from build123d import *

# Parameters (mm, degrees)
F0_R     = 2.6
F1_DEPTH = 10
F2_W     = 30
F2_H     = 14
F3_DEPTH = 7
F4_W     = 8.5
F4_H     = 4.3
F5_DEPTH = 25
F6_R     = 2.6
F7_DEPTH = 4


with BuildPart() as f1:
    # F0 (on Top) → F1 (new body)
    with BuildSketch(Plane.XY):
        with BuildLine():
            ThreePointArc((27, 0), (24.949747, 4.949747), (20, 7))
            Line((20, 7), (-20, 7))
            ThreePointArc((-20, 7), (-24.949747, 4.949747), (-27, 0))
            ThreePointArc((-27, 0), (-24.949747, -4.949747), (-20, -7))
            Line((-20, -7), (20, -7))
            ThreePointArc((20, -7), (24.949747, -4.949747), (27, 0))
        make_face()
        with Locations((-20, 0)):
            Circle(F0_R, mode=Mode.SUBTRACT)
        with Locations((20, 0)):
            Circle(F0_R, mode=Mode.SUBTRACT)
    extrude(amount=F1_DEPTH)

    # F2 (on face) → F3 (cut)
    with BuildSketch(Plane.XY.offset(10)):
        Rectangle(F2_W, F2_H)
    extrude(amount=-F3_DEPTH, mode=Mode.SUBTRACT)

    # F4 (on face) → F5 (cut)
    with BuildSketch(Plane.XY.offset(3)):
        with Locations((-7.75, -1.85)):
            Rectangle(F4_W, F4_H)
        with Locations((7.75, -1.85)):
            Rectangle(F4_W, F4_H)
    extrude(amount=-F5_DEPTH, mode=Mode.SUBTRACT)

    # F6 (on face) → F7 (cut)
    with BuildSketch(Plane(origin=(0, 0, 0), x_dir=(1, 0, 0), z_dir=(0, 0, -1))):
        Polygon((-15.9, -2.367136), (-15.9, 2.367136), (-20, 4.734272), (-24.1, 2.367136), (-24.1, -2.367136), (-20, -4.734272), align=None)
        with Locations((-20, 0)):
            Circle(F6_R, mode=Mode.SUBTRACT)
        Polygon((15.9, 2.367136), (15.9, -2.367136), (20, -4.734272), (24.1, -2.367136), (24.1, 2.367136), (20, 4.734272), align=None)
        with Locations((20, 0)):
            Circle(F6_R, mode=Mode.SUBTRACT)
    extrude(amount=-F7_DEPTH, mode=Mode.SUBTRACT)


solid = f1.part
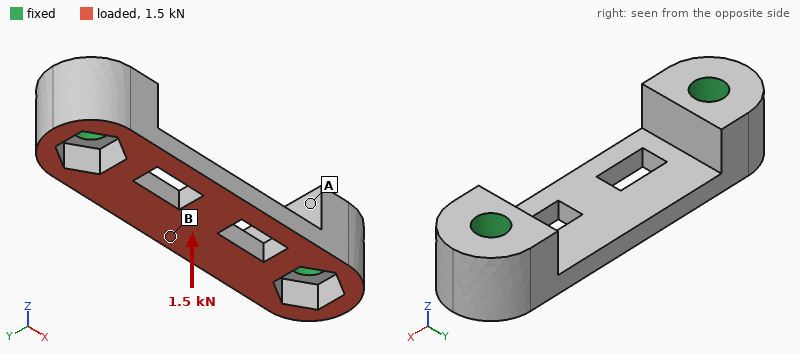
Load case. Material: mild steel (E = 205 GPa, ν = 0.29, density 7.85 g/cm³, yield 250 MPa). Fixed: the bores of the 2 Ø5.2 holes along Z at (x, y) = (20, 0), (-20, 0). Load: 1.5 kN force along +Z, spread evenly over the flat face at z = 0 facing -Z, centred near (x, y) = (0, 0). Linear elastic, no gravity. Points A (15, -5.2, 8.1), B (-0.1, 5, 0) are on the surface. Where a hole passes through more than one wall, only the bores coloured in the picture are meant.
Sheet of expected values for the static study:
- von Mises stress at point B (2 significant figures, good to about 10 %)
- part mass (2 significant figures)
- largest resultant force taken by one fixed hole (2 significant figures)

100 MPa
26 g
850 N
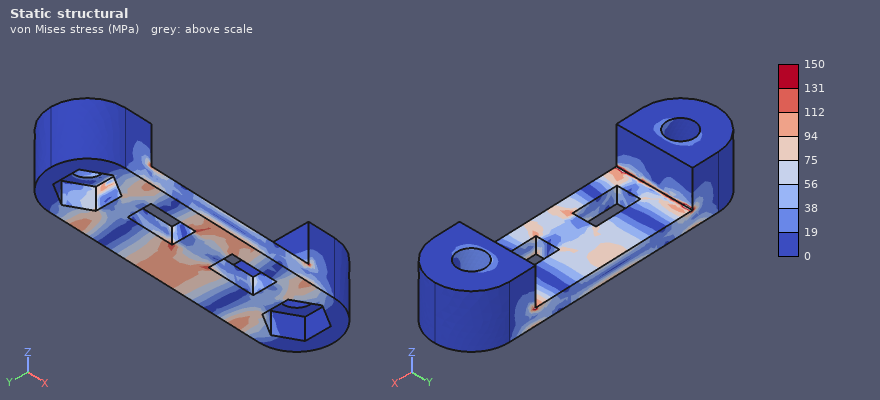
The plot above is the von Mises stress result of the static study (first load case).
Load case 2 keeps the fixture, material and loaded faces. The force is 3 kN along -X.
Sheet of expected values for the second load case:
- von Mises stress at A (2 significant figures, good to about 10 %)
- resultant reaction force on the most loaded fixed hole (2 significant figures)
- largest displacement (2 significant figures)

16 MPa
1.5 kN
5.4 µm
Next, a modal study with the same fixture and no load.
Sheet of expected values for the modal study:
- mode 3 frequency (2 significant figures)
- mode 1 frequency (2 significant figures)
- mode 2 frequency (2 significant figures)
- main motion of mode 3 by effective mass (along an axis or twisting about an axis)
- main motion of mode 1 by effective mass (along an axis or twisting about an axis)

21 kHz
13 kHz
19 kHz
along Y
along Z
